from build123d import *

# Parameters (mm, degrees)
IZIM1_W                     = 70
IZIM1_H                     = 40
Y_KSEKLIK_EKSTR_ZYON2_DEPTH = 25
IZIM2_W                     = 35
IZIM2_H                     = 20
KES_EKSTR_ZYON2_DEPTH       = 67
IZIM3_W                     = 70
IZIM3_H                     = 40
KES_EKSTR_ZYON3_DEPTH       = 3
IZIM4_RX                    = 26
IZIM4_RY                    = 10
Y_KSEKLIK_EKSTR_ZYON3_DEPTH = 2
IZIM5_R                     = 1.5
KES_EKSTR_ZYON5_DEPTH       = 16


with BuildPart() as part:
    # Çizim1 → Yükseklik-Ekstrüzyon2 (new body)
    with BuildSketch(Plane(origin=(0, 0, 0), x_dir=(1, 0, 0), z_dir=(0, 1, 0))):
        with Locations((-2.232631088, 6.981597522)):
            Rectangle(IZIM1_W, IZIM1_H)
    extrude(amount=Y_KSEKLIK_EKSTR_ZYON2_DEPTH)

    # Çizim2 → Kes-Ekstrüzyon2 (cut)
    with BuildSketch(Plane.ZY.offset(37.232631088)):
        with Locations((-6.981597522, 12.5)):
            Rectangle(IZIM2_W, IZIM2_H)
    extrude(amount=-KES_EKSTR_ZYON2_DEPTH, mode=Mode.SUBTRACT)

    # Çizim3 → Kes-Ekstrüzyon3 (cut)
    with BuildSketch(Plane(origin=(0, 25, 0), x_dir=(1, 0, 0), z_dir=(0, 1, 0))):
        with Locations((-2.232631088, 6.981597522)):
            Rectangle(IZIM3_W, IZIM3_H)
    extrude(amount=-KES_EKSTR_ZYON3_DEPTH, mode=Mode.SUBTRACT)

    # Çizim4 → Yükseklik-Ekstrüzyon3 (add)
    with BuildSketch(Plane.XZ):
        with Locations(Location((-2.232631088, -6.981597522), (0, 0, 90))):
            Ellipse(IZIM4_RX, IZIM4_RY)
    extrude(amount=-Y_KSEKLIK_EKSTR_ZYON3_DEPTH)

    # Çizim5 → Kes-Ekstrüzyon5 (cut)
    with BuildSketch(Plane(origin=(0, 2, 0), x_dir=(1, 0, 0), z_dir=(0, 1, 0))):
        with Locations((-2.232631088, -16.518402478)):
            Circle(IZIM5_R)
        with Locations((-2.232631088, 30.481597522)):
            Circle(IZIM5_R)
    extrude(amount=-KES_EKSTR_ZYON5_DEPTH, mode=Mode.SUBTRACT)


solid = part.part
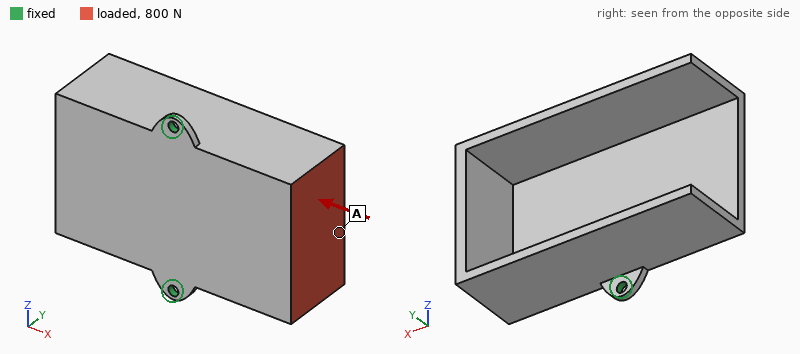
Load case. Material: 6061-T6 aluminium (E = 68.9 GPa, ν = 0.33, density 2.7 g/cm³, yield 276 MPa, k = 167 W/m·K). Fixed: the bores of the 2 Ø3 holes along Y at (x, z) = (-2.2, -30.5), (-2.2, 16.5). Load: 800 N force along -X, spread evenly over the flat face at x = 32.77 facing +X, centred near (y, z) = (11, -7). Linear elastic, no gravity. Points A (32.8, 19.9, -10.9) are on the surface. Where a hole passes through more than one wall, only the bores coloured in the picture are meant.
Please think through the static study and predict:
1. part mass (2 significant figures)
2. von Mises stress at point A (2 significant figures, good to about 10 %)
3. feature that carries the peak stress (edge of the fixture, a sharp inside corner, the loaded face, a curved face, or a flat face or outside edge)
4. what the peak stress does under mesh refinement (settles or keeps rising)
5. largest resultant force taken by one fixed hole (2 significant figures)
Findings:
43 g
32 MPa
edge of the fixture
keeps rising
400 N
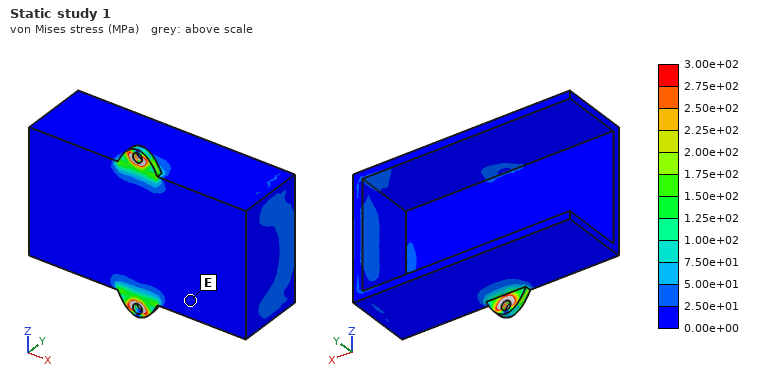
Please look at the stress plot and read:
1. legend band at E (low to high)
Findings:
0.00e+00 to 2.50e+01 MPa
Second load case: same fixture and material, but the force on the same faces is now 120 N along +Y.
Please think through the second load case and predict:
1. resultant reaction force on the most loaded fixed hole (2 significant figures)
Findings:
63 N
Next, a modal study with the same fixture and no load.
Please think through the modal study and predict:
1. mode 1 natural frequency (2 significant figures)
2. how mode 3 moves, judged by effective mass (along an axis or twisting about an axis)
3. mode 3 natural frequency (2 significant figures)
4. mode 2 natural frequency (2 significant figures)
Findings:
750 Hz
along Y
2600 Hz
2100 Hz
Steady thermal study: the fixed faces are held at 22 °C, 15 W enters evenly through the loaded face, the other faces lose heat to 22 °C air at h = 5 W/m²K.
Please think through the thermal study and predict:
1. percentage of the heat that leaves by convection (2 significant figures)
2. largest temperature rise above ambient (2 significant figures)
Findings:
6.1 %
29 K
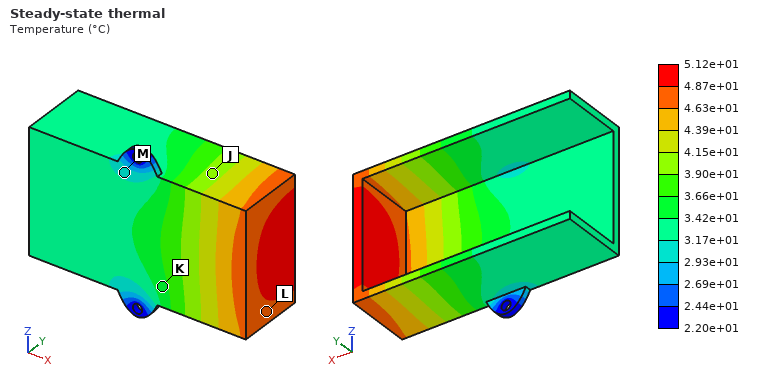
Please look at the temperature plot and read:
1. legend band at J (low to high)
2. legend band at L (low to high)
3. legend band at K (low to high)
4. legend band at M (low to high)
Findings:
3.90e+01 to 4.15e+01 °C
4.63e+01 to 4.87e+01 °C
3.42e+01 to 3.66e+01 °C
2.93e+01 to 3.17e+01 °C
